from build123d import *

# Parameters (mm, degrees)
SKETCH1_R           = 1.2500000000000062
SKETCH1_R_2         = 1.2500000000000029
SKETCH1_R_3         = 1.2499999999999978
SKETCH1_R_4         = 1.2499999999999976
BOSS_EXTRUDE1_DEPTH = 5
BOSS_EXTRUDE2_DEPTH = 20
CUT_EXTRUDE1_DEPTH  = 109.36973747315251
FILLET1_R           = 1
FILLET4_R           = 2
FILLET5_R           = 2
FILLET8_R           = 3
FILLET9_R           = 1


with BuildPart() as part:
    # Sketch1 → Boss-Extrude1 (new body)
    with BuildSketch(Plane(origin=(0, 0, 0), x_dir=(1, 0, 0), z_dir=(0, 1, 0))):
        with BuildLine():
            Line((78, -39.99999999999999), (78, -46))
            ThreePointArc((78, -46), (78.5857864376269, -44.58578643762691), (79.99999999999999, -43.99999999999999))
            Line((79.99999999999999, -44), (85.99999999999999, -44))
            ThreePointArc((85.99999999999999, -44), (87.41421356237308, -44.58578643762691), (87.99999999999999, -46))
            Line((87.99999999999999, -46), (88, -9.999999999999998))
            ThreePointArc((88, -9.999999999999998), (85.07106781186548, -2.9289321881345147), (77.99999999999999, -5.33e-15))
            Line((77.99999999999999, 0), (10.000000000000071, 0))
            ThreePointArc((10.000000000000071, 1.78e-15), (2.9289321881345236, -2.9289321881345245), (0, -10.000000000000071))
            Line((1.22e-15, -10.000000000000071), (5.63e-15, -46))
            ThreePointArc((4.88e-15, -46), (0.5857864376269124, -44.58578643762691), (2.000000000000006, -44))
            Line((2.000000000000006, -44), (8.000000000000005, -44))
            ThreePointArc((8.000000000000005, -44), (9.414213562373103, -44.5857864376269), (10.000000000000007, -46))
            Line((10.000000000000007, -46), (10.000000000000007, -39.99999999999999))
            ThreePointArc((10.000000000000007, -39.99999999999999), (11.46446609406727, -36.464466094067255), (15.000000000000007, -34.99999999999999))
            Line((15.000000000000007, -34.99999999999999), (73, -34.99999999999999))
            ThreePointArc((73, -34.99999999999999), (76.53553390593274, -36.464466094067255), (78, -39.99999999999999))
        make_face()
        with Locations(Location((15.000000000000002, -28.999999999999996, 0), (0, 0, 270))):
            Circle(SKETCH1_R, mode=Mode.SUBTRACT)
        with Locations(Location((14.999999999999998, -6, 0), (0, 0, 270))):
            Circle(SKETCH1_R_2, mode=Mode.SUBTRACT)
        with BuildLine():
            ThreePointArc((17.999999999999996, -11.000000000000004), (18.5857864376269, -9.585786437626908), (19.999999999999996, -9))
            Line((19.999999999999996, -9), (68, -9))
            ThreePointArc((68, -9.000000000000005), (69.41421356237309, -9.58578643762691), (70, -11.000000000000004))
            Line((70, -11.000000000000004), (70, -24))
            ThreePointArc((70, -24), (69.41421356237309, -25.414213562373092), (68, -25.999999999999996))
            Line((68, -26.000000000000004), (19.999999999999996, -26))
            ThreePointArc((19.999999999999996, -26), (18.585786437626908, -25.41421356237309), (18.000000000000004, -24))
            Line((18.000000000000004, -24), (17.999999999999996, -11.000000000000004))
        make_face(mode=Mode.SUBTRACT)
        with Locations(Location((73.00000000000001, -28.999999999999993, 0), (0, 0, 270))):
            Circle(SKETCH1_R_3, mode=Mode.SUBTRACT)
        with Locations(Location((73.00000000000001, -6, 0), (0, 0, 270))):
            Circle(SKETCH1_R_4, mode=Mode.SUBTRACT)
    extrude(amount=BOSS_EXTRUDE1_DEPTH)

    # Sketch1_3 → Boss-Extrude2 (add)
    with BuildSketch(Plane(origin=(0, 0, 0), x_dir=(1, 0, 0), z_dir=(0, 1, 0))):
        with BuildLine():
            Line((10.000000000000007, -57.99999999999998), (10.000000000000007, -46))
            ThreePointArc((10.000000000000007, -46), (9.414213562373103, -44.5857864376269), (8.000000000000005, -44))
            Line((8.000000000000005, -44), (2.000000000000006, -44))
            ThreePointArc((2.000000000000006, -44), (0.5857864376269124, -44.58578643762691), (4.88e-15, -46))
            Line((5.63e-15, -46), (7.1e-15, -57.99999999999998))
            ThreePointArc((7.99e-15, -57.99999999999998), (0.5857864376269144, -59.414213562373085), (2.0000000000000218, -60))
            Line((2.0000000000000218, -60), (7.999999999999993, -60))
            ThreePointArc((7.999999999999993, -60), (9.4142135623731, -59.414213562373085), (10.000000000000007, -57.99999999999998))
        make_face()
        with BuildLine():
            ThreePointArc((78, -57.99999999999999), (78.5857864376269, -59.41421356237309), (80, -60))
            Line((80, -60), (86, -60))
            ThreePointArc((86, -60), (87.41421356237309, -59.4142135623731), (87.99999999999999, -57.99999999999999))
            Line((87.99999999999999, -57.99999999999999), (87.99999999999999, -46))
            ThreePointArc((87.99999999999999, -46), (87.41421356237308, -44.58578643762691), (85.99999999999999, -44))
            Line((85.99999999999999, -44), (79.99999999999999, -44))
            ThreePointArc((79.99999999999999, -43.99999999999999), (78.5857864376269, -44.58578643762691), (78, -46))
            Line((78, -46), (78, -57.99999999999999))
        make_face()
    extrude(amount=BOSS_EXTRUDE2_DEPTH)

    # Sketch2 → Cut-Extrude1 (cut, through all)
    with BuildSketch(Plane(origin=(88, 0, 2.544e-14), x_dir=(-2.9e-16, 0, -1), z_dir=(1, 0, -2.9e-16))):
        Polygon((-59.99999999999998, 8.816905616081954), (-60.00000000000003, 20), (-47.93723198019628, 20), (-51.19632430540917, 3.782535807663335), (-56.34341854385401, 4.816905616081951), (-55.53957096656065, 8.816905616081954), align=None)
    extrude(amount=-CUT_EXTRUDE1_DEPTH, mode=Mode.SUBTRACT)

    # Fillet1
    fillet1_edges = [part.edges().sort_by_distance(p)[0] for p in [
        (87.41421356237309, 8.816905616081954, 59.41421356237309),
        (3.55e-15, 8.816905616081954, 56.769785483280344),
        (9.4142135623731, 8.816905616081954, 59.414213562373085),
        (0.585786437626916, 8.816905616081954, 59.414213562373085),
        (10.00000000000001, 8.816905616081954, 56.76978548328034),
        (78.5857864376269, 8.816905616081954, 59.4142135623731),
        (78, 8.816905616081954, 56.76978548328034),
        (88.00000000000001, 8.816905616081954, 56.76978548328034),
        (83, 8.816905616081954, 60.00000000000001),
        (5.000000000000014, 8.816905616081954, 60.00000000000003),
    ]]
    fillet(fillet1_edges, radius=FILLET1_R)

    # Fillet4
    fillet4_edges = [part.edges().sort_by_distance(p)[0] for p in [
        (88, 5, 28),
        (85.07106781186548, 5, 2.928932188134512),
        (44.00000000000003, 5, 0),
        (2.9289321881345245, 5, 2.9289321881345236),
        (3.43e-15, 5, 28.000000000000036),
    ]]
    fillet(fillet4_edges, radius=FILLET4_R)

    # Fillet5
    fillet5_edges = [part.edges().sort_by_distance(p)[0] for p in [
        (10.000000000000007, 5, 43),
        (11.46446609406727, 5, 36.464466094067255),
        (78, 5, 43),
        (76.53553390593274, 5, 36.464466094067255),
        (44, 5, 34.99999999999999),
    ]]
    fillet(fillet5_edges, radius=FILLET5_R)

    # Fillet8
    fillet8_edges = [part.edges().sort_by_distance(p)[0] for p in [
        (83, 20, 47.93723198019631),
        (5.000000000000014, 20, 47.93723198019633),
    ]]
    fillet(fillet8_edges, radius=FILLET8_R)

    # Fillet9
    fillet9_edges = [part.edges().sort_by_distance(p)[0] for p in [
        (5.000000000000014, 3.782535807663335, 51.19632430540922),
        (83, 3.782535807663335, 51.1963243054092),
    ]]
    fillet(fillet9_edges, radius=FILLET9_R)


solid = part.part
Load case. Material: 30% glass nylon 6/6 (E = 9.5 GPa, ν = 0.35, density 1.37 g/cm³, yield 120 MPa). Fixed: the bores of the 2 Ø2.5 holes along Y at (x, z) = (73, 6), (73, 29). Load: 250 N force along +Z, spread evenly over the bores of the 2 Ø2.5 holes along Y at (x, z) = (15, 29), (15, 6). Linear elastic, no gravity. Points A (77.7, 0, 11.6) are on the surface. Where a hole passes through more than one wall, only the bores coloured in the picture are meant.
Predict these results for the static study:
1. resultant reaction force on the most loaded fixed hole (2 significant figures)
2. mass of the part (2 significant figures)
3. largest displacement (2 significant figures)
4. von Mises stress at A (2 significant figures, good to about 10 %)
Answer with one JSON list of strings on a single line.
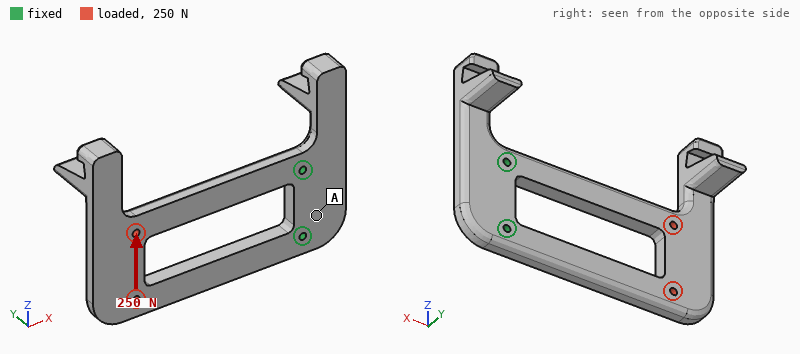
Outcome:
["550 N", "20 g", "1.0 mm", "8.1 MPa"]
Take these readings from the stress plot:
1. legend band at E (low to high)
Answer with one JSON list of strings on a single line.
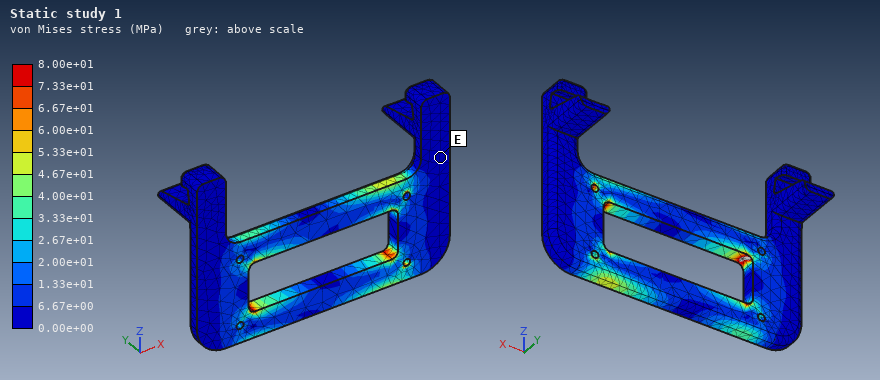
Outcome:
["0.00e+00 to 6.67e+00 MPa"]
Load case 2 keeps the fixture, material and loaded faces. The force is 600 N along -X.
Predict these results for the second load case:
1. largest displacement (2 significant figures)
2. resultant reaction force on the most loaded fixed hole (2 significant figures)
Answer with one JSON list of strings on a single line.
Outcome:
["59 µm", "300 N"]
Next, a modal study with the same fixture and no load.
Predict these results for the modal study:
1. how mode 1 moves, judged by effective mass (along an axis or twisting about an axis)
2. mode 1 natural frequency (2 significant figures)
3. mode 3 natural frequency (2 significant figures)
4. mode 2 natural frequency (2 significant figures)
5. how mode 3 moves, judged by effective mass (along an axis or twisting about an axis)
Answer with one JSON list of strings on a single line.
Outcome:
["along Y", "230 Hz", "820 Hz", "620 Hz", "along Z"]
